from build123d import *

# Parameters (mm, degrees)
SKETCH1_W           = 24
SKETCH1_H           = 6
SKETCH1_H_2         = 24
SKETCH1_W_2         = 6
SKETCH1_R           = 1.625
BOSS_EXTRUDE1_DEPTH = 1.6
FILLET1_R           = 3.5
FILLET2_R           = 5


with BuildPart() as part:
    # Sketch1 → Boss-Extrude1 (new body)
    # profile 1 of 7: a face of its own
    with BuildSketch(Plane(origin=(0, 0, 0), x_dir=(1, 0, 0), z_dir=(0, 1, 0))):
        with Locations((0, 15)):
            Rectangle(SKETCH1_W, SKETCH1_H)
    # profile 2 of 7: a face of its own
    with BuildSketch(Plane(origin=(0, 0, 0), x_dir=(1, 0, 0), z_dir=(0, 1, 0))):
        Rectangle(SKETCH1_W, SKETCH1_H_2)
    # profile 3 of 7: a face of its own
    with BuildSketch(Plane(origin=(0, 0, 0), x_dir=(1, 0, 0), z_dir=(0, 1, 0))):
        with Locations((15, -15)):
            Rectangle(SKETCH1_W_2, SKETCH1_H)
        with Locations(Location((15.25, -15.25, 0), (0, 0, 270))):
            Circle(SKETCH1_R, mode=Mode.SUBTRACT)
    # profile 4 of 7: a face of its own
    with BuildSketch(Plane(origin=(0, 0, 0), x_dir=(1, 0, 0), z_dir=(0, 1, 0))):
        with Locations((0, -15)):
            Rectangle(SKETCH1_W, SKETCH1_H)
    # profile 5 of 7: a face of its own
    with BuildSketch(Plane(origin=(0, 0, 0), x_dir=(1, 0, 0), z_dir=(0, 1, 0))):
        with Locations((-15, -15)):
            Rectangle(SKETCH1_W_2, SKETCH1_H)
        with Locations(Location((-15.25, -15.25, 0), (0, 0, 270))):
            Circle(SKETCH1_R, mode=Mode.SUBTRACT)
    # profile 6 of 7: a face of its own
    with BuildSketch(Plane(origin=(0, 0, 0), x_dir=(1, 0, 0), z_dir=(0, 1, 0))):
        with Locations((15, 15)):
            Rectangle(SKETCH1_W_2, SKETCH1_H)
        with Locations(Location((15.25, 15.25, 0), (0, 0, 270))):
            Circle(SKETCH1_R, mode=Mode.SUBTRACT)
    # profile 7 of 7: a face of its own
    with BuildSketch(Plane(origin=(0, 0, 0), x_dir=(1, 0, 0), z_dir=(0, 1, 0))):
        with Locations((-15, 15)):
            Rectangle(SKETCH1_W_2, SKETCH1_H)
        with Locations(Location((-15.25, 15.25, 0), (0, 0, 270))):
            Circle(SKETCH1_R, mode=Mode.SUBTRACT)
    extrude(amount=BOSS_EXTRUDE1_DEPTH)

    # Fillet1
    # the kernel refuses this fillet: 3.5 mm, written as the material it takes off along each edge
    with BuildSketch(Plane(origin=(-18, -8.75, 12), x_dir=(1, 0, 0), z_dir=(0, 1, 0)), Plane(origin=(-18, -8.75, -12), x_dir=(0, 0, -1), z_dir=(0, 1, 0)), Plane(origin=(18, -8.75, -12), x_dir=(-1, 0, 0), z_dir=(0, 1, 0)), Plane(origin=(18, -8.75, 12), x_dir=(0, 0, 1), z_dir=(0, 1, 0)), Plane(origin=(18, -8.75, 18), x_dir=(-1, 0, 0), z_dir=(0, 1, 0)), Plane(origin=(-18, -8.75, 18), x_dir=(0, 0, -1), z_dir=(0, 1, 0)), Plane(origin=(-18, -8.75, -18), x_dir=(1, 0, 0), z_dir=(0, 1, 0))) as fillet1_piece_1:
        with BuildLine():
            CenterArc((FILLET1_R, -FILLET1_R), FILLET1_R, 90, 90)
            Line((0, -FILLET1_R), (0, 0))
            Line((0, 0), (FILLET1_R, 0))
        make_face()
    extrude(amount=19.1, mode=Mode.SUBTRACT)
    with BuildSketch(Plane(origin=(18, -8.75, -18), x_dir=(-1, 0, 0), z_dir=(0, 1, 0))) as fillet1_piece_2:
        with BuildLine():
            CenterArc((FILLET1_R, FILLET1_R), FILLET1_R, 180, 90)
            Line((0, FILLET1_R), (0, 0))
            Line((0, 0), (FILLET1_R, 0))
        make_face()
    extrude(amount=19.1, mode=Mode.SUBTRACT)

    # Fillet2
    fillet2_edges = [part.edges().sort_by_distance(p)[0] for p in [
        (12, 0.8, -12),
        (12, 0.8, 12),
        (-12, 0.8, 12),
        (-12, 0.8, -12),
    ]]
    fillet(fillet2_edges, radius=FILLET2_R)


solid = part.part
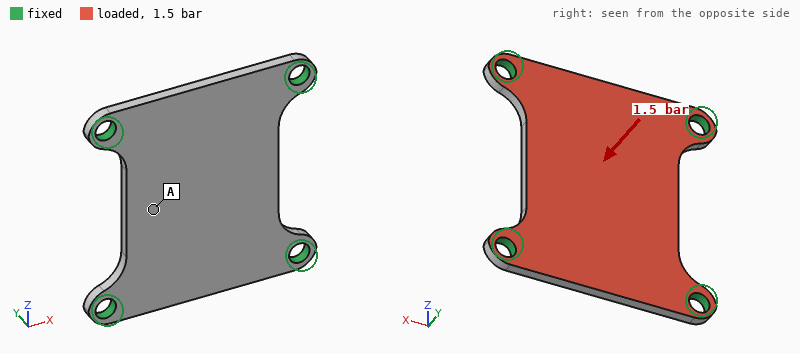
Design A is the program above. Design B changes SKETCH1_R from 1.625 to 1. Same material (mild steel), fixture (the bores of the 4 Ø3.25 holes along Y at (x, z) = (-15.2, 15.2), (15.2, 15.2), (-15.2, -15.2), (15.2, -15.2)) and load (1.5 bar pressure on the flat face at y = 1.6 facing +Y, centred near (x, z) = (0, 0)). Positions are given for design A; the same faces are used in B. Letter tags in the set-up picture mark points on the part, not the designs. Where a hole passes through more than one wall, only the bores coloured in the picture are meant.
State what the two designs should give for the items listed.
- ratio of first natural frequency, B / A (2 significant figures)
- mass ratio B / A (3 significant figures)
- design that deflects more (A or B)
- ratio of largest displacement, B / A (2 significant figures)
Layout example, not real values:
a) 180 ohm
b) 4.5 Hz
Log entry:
a) 0.91
b) 1.02
c) B
d) 1.2
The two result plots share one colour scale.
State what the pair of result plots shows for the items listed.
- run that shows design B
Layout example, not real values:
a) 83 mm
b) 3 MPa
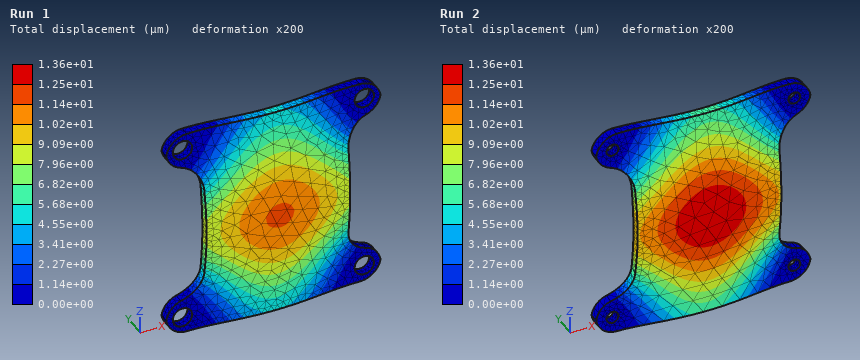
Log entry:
a) Run 2
